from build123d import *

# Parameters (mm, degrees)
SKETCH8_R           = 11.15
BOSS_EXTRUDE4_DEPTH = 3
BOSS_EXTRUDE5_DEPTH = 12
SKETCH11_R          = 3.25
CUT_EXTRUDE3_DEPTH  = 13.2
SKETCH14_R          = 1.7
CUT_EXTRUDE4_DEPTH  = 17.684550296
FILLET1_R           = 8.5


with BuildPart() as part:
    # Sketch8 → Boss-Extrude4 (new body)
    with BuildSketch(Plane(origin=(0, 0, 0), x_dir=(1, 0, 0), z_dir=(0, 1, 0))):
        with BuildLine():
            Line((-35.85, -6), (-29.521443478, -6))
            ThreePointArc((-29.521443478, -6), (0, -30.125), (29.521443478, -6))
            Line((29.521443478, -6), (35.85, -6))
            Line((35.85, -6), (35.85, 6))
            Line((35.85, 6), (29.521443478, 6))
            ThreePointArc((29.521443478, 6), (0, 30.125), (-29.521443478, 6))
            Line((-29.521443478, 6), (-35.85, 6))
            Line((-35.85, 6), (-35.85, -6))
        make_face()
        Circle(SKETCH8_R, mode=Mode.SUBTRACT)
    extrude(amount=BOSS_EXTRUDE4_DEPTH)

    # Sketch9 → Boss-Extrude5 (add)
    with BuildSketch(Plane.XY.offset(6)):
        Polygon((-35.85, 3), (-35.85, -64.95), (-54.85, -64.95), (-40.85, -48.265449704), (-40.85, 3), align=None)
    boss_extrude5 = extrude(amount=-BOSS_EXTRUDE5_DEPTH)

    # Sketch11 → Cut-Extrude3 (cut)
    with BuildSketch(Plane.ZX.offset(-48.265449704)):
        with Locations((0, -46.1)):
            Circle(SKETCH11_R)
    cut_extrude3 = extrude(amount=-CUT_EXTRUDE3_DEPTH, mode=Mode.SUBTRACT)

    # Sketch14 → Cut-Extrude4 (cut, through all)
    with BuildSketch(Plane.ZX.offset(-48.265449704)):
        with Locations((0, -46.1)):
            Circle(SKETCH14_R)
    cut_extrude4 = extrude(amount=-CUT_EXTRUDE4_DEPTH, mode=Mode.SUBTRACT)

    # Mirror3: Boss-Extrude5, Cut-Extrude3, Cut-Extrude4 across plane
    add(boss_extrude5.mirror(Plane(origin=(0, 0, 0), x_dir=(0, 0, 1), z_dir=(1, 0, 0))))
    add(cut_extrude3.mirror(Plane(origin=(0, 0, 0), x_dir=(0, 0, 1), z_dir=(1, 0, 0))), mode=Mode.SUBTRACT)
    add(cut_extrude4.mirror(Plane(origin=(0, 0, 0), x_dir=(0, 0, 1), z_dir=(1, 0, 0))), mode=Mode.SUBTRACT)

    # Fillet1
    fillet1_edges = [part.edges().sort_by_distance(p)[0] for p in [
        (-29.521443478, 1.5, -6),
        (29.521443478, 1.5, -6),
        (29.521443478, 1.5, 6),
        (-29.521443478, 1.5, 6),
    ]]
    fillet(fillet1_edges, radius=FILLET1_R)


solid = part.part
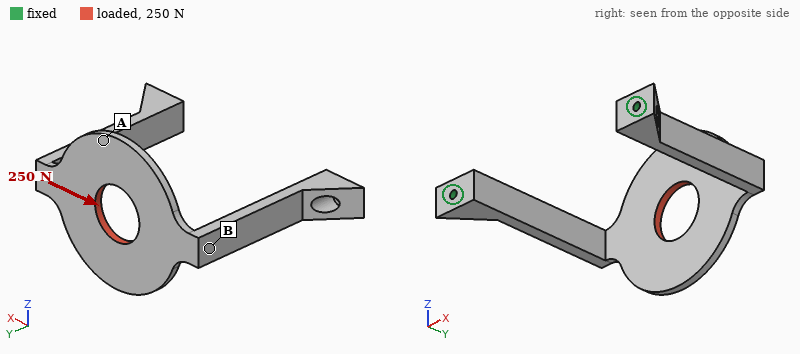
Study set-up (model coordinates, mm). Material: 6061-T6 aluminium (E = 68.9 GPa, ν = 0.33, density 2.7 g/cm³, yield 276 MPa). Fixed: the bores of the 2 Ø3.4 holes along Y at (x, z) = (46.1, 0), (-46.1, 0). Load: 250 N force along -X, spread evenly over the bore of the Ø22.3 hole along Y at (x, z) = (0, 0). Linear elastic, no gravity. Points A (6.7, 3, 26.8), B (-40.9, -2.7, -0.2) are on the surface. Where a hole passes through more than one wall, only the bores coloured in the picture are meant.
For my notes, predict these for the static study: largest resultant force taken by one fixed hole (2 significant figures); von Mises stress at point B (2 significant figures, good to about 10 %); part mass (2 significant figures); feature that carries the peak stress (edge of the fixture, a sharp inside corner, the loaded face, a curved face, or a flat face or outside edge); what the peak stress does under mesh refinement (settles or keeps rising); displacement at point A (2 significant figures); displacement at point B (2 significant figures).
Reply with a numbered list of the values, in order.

1. 140 N
2. 30 MPa
3. 49 g
4. edge of the fixture
5. keeps rising
6. 0.53 mm
7. 0.49 mm
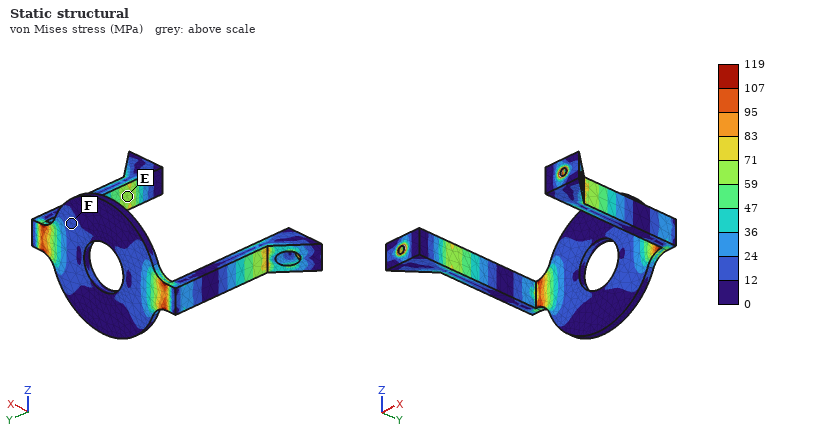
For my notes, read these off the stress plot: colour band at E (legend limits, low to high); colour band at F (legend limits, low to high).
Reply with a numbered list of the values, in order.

1. 59 to 71 MPa
2. 12 to 24 MPa
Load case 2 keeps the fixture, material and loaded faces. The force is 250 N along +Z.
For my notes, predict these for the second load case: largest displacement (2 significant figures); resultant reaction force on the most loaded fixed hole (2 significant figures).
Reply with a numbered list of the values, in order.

1. 0.48 mm
2. 130 N
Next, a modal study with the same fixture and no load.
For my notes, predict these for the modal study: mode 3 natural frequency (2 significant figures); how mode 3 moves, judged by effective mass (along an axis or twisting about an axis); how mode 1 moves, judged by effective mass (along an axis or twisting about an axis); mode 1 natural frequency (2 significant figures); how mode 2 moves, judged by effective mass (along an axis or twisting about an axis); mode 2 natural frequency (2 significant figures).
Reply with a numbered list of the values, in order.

1. 1300 Hz
2. twisting about Y
3. along X
4. 660 Hz
5. along Z
6. 720 Hz
